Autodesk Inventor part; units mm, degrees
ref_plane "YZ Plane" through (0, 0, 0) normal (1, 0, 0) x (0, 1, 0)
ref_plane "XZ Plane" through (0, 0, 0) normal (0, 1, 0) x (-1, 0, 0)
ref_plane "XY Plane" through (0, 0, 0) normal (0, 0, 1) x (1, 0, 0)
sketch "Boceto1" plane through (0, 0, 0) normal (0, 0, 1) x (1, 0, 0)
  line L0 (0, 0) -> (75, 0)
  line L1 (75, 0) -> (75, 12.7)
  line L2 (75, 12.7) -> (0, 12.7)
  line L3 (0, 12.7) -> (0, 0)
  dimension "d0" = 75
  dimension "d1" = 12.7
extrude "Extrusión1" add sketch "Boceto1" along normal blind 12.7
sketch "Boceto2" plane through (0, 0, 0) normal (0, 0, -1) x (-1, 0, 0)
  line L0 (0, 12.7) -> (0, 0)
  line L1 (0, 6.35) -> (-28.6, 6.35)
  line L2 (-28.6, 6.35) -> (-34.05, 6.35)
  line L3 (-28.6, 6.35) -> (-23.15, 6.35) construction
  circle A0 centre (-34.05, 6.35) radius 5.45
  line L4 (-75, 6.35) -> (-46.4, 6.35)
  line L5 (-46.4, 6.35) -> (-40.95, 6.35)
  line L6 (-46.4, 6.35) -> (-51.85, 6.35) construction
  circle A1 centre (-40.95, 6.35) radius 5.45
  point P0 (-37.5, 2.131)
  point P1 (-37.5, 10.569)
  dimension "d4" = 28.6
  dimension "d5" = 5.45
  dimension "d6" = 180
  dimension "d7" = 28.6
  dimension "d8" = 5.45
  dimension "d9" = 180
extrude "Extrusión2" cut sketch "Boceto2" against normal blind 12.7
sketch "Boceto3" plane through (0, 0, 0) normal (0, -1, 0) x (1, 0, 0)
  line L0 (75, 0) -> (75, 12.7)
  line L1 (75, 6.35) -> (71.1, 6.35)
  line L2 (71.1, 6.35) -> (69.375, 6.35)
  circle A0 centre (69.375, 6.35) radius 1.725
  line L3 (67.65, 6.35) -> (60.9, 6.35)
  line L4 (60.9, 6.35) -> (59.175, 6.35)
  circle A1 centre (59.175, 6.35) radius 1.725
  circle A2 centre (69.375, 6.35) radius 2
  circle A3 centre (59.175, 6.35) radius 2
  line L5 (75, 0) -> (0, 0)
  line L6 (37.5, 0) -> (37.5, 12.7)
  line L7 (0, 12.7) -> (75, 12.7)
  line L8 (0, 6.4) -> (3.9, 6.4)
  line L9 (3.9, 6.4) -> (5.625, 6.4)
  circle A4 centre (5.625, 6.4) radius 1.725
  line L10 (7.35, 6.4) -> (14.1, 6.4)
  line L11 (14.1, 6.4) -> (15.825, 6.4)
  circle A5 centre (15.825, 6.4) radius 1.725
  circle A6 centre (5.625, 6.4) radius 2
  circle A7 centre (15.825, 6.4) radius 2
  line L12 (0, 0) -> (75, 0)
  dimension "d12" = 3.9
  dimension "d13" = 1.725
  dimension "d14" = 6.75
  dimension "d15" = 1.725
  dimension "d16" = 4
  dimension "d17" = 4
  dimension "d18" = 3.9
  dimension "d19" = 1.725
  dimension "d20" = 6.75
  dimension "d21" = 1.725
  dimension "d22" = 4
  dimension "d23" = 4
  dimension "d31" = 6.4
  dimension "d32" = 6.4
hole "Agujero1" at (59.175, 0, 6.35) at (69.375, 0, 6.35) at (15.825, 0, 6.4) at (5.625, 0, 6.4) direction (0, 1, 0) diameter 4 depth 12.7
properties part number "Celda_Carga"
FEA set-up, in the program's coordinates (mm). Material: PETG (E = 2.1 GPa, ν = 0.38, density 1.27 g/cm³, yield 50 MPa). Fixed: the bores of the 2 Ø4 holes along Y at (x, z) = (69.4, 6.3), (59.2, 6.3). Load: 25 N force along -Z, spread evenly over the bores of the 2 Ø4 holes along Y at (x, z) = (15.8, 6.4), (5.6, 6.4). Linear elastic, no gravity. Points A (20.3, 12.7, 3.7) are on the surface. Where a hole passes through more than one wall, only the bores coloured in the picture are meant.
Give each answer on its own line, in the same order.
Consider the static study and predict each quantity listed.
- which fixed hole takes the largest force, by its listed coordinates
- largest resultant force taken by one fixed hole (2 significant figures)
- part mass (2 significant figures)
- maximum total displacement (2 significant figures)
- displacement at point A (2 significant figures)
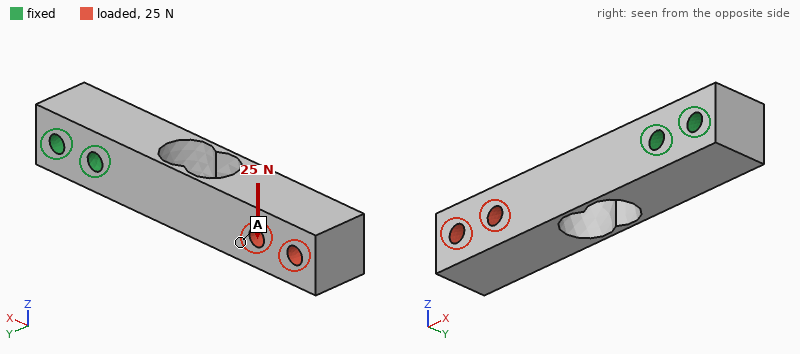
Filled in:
(59.2, 6.3)
80 N
12 g
0.90 mm
0.46 mm
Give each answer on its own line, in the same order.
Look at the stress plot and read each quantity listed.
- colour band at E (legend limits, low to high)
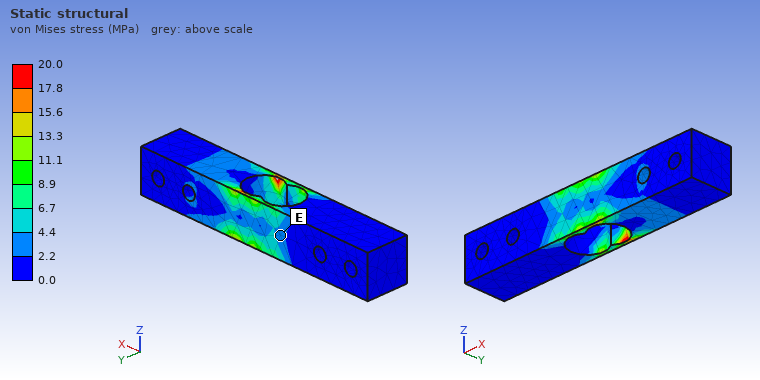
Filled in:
2.2 to 4.4 MPa
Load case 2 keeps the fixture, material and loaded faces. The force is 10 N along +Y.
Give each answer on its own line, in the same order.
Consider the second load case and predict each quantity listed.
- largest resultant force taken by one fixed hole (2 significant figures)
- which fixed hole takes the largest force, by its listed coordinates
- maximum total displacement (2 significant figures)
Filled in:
15 N
(59.2, 6.3)
0.45 mm
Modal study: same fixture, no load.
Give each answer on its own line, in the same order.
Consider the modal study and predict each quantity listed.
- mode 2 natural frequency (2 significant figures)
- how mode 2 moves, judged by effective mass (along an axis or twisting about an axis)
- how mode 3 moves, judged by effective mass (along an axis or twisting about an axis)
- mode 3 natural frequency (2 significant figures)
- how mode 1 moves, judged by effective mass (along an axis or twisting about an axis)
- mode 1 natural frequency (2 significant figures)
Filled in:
450 Hz
along Z
twisting about X
1600 Hz
along Y
340 Hz
